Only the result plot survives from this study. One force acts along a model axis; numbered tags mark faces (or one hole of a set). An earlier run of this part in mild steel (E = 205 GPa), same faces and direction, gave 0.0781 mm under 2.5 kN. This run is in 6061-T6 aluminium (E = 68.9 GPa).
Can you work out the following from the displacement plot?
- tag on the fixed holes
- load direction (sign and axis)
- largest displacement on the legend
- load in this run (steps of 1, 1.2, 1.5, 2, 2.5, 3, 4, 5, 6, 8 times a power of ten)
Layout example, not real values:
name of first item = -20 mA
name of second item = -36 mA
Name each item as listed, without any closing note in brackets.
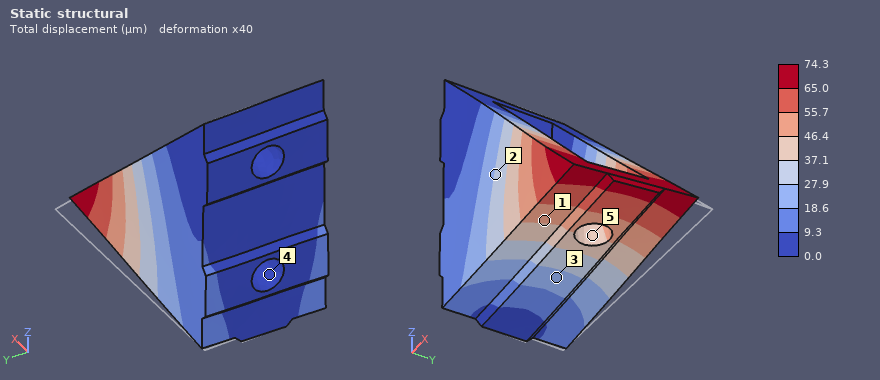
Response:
tag on the fixed holes = 4
load direction = -Y
largest displacement on the legend = 74.3 µm
load in this run = 800 N
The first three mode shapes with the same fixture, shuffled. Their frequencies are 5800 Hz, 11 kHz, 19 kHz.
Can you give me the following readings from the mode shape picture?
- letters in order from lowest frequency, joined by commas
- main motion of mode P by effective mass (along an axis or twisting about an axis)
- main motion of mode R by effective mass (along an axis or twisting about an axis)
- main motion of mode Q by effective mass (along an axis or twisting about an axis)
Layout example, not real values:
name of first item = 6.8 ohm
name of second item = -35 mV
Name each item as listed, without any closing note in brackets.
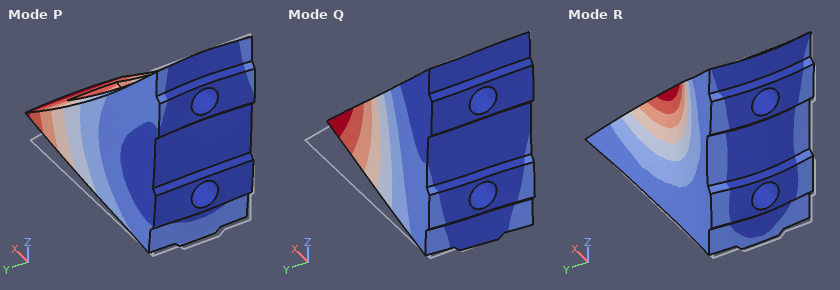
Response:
letters in order from lowest frequency, joined by commas = Q, P, R
main motion of mode P by effective mass = along Z
main motion of mode R by effective mass = along X
main motion of mode Q by effective mass = along Y
